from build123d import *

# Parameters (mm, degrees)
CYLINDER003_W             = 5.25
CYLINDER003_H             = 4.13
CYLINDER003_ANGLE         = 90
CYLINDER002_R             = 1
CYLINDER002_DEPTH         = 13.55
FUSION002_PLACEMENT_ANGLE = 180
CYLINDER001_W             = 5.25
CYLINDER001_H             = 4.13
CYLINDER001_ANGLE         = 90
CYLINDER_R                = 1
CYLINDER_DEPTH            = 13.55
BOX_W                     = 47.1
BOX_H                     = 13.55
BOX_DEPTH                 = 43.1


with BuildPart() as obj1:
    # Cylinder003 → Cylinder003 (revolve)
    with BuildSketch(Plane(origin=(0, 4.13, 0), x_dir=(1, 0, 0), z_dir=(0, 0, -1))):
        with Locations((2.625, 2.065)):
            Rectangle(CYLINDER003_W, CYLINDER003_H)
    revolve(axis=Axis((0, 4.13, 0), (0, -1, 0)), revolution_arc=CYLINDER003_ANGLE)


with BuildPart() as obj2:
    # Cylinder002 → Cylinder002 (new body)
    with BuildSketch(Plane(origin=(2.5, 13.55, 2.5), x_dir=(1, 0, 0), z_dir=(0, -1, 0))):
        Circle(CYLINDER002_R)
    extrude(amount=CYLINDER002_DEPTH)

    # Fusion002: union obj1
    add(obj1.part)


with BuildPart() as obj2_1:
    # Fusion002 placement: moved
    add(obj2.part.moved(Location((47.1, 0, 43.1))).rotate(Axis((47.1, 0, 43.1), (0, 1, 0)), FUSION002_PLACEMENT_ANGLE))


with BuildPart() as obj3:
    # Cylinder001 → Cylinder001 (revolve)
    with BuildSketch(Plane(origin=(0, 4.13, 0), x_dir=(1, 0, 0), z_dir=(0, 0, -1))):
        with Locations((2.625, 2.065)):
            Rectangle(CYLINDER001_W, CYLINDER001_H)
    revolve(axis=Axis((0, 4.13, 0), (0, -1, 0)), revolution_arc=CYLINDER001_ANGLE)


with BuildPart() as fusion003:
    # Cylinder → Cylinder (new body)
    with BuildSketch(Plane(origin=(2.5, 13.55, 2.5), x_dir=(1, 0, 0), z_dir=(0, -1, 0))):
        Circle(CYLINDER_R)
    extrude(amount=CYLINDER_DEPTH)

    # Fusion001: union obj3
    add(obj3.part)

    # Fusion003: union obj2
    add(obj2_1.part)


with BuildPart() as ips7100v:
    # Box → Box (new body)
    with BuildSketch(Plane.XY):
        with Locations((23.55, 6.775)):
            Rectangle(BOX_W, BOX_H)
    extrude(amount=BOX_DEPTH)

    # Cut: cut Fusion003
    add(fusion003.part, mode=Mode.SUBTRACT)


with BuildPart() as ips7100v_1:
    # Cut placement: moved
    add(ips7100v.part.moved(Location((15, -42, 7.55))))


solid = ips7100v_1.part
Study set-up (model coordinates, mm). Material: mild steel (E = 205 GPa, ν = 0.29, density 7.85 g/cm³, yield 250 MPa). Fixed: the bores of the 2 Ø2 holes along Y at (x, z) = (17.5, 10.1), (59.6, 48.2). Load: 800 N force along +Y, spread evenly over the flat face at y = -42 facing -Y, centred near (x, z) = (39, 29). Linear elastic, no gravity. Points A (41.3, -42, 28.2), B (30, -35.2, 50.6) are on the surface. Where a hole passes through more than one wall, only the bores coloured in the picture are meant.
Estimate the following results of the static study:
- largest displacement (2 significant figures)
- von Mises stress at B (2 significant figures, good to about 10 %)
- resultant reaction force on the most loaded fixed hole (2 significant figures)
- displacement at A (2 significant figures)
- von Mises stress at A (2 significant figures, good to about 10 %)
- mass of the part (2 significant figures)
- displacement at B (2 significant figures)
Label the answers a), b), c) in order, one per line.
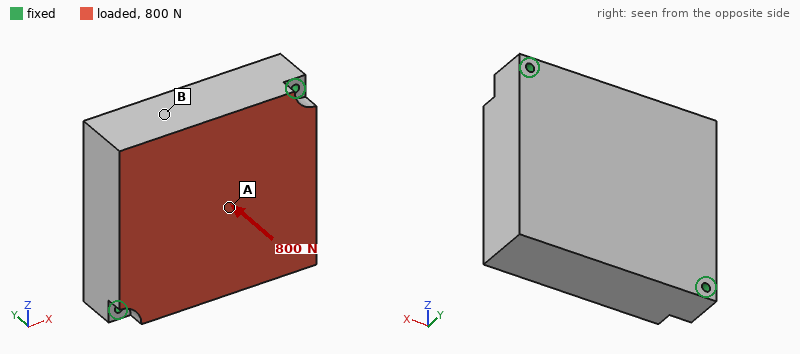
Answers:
a) 2.3 µm
b) 2.2 MPa
c) 440 N
d) 1.5 µm
e) 5.4 MPa
f) 210 g
g) 1.8 µm
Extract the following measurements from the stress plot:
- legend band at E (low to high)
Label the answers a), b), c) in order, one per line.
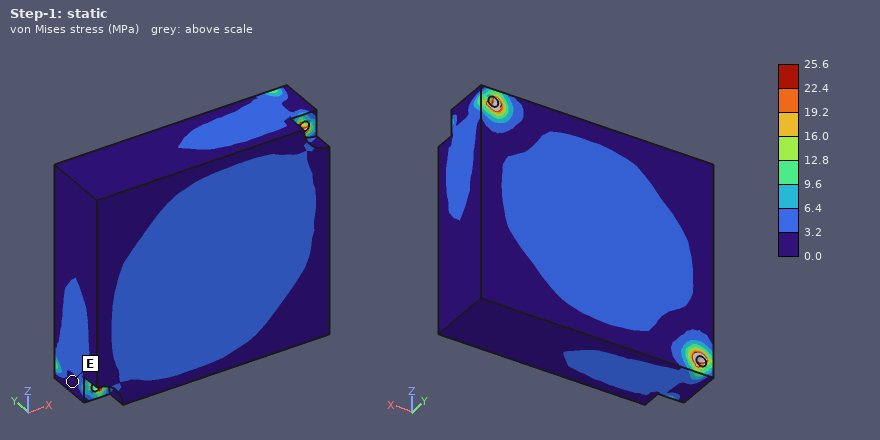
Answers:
a) 0.0 to 3.2 MPa
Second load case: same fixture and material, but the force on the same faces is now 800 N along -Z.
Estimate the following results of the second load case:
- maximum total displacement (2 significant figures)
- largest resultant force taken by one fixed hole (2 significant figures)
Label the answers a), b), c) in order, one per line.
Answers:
a) 5.2 µm
b) 410 N
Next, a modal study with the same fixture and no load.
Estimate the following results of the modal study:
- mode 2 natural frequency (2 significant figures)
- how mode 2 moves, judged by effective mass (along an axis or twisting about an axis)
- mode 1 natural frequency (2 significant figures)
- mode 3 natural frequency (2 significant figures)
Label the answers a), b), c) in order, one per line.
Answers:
a) 7900 Hz
b) along Y
c) 4500 Hz
d) 13 kHz
